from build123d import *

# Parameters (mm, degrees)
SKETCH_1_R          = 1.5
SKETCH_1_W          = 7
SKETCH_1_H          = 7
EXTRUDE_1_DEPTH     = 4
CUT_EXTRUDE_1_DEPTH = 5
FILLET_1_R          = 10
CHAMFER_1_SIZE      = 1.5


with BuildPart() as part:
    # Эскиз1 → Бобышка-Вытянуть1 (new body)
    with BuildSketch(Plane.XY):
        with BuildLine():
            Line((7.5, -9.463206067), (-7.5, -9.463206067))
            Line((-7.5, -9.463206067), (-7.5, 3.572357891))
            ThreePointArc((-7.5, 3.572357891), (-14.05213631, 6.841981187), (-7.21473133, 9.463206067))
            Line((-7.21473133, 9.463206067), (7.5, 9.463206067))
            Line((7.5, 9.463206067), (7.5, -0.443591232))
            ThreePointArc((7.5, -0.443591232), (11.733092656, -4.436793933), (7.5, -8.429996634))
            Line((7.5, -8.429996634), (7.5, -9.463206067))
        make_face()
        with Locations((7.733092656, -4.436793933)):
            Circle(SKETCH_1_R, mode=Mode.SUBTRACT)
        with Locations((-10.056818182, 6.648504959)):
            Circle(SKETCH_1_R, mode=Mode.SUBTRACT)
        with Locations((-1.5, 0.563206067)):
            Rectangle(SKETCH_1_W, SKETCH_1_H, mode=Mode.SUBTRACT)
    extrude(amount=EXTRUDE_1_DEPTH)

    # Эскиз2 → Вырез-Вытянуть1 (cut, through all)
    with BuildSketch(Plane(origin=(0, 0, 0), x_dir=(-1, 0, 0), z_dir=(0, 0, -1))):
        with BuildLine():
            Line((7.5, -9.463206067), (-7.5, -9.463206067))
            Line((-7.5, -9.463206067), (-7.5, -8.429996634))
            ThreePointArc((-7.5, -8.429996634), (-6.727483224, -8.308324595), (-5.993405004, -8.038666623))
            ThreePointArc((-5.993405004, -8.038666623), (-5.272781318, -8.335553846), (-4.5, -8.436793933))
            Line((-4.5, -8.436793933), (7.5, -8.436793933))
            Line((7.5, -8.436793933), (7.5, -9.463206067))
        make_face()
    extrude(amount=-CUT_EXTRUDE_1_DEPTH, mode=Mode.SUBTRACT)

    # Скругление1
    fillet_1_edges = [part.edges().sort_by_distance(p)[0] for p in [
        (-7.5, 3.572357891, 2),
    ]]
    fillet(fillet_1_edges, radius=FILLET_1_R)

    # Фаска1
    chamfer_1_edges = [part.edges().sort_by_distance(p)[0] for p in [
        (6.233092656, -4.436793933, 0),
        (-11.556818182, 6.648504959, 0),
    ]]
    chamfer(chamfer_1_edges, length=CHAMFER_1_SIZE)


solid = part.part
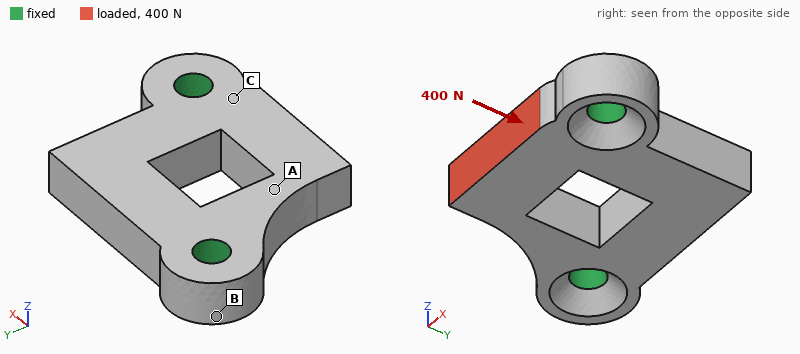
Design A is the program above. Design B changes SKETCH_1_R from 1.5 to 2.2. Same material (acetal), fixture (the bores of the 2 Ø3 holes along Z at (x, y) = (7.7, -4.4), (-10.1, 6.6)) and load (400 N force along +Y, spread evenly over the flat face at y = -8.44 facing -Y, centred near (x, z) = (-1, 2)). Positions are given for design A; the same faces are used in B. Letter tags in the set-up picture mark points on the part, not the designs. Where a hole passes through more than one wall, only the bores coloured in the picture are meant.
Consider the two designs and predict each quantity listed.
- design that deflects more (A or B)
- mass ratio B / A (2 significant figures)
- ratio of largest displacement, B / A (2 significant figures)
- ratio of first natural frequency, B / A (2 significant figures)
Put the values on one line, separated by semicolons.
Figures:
A; 0.93; 0.89; 1.1
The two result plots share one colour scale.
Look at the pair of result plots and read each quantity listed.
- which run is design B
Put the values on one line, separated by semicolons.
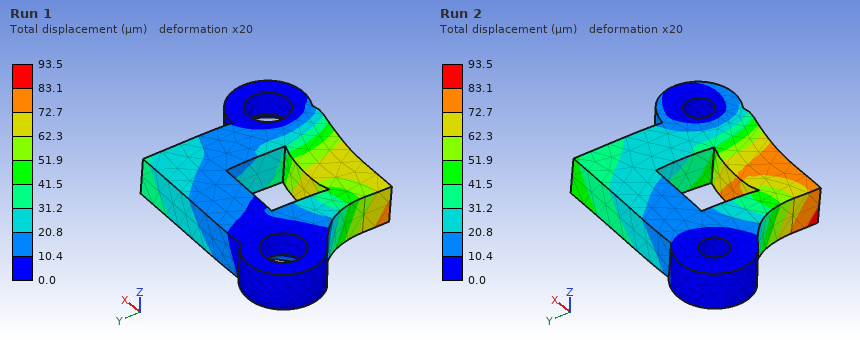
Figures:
Run 1
